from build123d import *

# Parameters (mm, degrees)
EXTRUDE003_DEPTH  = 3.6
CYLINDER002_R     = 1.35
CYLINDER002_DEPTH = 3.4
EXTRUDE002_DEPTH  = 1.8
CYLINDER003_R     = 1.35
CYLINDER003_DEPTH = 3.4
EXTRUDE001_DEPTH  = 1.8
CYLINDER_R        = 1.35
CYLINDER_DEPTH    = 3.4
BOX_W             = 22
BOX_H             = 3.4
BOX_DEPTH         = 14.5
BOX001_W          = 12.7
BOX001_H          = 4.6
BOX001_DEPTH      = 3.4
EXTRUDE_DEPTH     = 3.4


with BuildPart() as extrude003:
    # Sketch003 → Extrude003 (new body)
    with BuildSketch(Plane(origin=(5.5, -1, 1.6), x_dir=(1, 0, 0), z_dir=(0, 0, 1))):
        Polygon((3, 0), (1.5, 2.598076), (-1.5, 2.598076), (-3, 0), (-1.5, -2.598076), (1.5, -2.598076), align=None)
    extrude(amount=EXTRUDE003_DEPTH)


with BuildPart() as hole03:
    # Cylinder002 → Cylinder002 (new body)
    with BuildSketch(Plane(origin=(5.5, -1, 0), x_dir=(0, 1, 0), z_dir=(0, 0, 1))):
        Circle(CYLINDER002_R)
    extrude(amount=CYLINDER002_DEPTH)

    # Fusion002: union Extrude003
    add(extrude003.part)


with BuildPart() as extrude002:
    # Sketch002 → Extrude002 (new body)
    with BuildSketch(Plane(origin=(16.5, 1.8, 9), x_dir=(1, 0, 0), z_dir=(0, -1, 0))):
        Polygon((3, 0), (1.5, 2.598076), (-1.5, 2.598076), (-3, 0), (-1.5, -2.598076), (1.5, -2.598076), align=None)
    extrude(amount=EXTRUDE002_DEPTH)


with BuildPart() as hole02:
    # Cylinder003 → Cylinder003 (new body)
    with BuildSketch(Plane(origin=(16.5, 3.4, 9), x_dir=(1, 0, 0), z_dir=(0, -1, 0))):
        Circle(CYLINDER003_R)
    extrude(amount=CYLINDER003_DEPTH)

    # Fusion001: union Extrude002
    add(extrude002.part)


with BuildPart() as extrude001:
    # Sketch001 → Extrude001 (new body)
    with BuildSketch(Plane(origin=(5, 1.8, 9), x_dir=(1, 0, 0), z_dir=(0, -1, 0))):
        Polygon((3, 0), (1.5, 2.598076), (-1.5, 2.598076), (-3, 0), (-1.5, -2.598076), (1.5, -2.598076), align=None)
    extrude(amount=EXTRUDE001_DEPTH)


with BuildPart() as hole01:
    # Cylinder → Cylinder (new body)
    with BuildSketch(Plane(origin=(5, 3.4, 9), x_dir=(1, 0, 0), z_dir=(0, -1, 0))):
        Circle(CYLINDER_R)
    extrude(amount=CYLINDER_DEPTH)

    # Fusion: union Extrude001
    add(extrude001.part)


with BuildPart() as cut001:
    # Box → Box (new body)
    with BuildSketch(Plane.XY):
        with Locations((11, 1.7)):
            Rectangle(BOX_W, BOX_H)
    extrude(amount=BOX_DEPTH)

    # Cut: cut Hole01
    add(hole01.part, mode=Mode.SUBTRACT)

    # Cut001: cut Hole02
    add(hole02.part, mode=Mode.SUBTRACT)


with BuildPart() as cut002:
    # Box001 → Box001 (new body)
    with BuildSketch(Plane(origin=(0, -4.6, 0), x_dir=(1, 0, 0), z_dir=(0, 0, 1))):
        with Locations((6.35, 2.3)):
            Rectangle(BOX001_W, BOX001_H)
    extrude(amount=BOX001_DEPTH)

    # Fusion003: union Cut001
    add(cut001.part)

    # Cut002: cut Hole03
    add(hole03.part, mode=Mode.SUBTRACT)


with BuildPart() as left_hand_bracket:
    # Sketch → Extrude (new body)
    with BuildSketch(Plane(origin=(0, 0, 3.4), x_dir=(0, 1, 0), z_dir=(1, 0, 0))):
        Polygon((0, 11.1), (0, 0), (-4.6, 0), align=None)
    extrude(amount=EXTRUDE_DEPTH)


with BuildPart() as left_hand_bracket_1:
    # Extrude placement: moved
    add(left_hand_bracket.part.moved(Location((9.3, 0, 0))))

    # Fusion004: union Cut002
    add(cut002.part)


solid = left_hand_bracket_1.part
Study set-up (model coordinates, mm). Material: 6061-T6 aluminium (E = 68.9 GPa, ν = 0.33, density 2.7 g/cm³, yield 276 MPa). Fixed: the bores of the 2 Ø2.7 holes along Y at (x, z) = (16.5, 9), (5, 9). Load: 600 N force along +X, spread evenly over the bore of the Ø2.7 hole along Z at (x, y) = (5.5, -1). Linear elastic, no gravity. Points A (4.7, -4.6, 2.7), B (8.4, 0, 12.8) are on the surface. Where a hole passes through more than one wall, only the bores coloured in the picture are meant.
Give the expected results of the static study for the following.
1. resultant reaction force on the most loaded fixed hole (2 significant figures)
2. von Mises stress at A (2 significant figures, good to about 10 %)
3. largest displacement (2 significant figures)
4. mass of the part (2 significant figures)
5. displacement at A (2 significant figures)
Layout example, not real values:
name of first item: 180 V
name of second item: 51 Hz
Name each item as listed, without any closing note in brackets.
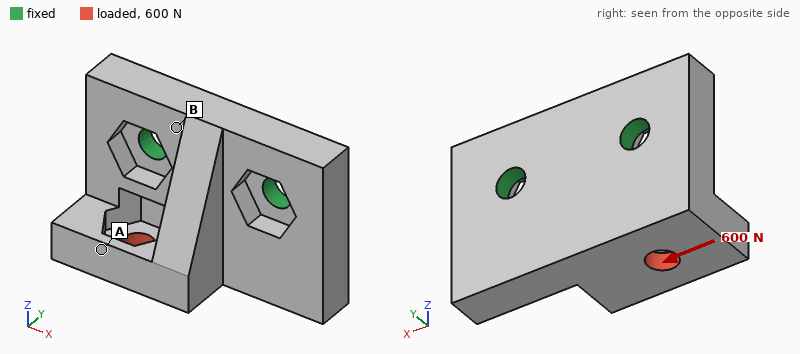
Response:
resultant reaction force on the most loaded fixed hole: 530 N
von Mises stress at A: 26 MPa
largest displacement: 19 µm
mass of the part: 3.3 g
displacement at A: 15 µm
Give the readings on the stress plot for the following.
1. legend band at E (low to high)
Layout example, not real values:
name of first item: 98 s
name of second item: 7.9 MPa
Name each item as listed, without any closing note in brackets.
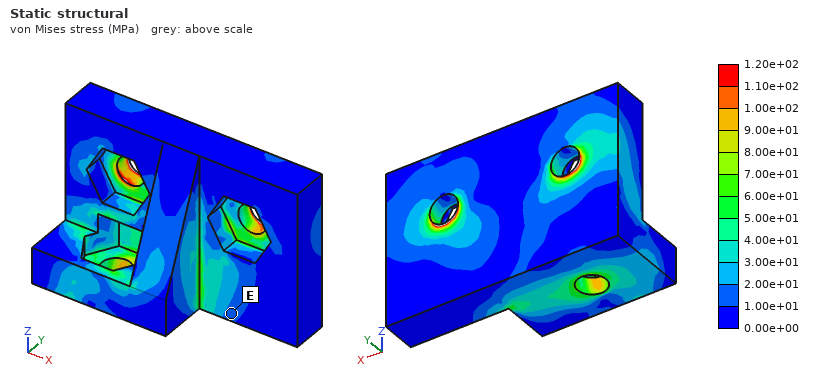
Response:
legend band at E: 1.00e+01 to 2.00e+01 MPa
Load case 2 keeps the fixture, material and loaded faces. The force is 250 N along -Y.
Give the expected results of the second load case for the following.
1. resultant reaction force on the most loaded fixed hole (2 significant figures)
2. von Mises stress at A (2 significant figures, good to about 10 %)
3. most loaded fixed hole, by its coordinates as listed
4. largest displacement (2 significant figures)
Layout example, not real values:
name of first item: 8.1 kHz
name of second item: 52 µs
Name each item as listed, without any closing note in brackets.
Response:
resultant reaction force on the most loaded fixed hole: 230 N
von Mises stress at A: 18 MPa
most loaded fixed hole, by its coordinates as listed: (5, 9)
largest displacement: 48 µm
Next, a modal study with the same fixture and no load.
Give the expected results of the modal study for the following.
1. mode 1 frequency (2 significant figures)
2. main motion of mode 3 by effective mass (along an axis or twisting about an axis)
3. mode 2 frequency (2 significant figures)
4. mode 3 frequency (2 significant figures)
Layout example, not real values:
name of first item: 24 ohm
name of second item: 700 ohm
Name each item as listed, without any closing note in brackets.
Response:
mode 1 frequency: 13 kHz
main motion of mode 3 by effective mass: along X
mode 2 frequency: 25 kHz
mode 3 frequency: 38 kHz
